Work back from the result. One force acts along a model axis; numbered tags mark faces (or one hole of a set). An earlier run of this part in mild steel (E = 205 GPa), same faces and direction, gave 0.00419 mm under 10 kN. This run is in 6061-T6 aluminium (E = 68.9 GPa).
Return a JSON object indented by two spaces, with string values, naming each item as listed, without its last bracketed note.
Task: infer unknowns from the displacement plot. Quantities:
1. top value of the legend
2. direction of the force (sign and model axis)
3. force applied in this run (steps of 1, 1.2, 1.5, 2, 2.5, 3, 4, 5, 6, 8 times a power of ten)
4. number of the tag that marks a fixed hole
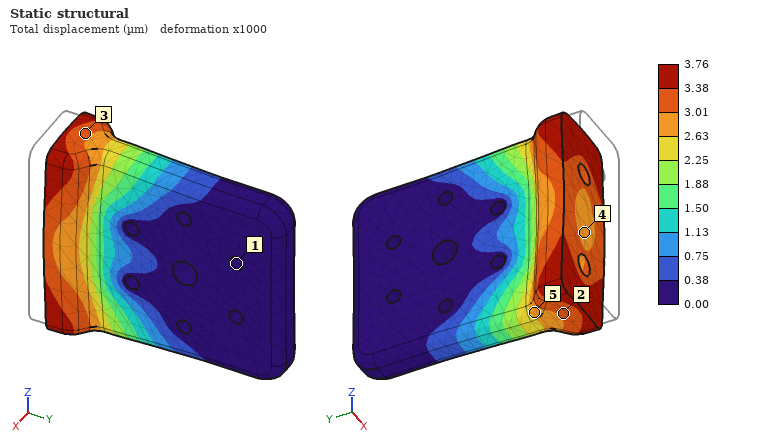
{
  "top value of the legend": "3.76 µm",
  "direction of the force": "+Y",
  "force applied in this run": "3 kN",
  "number of the tag that marks a fixed hole": "1"
}
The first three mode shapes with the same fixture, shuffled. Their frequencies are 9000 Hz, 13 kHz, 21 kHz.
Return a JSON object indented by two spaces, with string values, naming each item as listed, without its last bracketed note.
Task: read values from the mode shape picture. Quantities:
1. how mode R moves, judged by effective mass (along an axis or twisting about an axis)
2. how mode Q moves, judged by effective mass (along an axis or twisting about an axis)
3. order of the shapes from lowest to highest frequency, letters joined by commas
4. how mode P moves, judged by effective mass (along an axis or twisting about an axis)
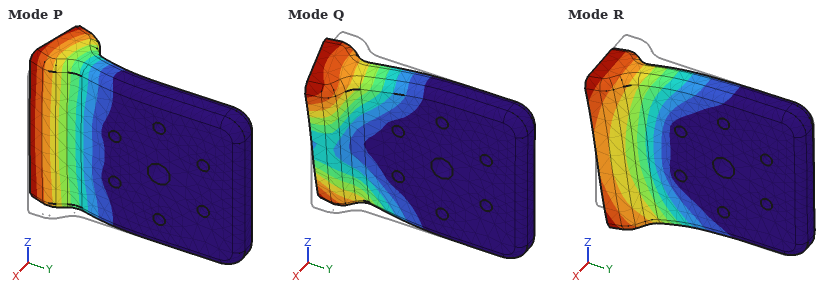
{
  "how mode R moves, judged by effective mass": "along Z",
  "how mode Q moves, judged by effective mass": "twisting about Y",
  "order of the shapes from lowest to highest frequency, letters joined by commas": "P, Q, R",
  "how mode P moves, judged by effective mass": "along X"
}
